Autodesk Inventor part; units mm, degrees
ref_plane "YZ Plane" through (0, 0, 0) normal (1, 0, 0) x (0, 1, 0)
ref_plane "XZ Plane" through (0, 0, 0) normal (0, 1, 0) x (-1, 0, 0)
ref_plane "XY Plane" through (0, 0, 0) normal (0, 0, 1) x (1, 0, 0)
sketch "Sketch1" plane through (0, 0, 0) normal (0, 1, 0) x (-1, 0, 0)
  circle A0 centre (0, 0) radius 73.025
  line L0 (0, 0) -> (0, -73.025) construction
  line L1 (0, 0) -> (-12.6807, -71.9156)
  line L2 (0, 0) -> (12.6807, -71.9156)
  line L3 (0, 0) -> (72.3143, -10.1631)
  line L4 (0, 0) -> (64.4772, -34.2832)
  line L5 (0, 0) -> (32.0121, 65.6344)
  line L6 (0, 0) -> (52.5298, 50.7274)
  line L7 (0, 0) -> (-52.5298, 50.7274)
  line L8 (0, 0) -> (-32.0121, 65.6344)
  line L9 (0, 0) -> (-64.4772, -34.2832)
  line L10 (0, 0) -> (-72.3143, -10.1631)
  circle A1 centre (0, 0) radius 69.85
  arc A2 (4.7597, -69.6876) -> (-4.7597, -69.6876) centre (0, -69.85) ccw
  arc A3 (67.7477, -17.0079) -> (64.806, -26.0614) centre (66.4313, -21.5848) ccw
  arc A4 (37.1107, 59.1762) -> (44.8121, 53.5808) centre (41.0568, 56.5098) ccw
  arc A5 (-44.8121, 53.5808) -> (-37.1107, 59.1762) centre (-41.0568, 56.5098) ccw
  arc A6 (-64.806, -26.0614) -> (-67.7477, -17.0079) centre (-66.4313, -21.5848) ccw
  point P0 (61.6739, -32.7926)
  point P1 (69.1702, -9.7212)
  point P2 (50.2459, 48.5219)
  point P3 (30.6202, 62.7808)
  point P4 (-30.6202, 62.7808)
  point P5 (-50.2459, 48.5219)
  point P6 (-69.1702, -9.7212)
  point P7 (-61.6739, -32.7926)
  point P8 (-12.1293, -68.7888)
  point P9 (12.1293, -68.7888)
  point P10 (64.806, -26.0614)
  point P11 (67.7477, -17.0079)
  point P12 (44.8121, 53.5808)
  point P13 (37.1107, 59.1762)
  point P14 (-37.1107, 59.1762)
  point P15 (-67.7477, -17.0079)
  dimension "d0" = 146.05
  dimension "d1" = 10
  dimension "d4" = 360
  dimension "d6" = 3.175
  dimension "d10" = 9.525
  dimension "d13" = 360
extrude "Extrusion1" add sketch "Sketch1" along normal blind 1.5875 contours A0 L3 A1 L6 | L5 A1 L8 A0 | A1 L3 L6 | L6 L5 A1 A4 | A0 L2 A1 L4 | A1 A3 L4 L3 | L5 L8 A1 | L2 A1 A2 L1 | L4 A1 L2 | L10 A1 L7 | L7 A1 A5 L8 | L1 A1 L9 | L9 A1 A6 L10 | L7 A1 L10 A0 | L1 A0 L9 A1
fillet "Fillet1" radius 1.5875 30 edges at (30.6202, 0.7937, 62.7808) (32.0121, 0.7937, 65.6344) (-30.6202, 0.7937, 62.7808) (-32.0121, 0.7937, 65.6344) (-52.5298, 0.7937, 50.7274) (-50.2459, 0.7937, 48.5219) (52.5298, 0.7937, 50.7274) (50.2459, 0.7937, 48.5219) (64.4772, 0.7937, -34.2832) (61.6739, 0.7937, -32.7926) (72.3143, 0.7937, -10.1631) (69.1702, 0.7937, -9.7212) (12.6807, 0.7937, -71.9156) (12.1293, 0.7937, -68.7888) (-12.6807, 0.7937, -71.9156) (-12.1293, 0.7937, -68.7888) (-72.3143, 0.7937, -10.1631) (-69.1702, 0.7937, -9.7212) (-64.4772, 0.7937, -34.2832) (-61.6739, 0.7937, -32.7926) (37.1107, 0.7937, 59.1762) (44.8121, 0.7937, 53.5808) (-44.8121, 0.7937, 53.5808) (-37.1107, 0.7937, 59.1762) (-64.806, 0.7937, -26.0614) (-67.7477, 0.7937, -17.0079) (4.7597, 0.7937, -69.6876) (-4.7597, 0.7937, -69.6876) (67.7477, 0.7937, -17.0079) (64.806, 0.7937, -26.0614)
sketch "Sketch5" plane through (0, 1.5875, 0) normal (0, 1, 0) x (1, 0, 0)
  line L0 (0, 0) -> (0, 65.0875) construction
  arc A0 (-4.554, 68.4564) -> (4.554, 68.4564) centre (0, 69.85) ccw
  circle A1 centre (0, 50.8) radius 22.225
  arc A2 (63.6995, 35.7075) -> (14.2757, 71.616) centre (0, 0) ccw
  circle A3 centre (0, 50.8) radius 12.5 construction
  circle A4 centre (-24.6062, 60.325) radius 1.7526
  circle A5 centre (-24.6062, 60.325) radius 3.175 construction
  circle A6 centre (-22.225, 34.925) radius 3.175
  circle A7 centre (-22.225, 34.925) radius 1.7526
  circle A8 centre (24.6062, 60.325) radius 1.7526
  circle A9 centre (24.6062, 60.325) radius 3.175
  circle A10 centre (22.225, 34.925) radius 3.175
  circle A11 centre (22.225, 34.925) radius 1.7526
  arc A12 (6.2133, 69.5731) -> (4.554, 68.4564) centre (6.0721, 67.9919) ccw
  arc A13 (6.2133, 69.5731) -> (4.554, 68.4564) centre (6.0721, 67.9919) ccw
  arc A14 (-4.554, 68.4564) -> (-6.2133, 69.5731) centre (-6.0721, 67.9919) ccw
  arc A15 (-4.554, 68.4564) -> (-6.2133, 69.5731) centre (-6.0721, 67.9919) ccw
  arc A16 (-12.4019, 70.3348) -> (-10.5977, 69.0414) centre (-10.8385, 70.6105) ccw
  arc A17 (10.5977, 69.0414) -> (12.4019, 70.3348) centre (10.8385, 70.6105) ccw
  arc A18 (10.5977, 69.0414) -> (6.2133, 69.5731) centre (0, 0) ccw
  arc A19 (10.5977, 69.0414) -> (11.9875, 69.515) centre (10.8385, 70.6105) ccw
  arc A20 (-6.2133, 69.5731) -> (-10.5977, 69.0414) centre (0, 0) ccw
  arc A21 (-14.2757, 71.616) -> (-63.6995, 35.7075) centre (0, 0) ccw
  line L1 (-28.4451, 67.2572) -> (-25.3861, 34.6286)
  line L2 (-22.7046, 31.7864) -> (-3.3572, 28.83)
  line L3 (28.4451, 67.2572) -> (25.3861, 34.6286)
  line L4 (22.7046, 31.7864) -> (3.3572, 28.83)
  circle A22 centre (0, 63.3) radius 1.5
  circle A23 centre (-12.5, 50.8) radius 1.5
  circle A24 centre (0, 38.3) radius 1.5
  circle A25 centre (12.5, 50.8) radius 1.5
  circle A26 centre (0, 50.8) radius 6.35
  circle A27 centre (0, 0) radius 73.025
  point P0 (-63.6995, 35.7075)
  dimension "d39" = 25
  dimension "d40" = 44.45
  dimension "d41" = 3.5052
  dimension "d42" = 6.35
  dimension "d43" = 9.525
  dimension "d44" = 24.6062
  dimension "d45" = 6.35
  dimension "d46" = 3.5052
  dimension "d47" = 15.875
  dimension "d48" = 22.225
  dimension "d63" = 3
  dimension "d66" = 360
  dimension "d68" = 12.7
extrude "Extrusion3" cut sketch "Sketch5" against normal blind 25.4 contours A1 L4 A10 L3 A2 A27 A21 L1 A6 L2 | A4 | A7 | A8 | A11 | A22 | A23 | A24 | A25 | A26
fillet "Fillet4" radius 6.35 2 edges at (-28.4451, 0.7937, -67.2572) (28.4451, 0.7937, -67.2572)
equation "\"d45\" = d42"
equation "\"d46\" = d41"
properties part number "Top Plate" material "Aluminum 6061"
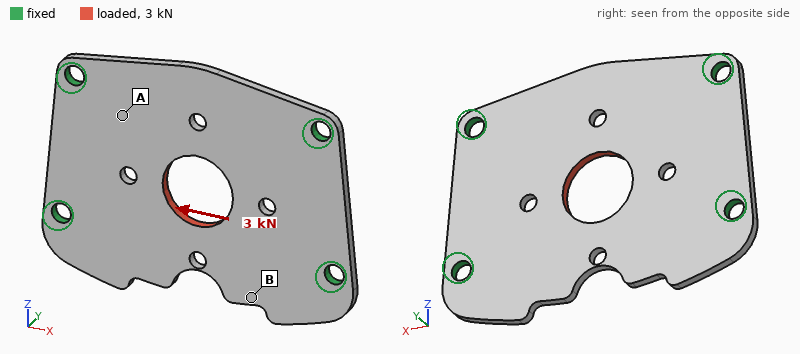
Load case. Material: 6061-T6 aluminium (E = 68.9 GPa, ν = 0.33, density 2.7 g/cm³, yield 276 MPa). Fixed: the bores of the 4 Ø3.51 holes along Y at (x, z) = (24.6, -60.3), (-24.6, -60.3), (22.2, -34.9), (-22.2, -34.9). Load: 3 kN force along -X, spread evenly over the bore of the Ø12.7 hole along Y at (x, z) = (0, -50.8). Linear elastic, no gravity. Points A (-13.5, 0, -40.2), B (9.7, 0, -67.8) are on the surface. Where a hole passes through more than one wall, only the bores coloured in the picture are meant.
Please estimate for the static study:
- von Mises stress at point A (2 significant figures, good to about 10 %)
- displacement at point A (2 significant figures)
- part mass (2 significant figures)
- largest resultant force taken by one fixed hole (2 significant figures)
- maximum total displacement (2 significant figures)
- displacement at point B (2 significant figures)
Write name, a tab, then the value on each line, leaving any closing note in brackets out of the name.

von Mises stress at point A	36 MPa
displacement at point A	6.4 µm
part mass	8.0 g
largest resultant force taken by one fixed hole	880 N
maximum total displacement	15 µm
displacement at point B	6.8 µm
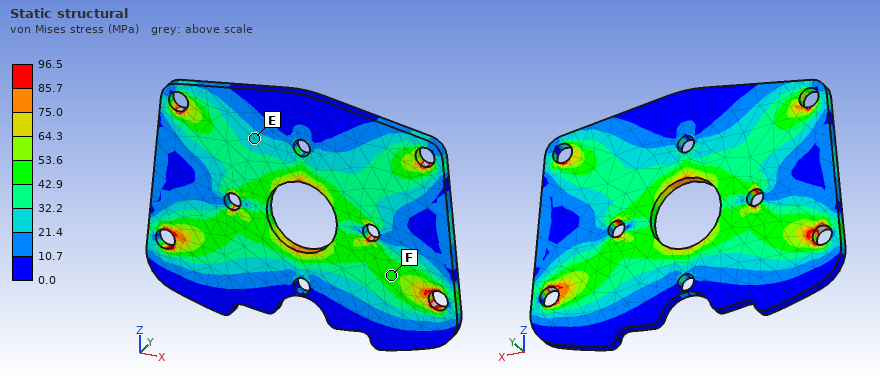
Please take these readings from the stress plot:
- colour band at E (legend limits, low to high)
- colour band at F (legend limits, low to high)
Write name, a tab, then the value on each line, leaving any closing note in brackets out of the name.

colour band at E	21.4 to 32.2 MPa
colour band at F	42.9 to 53.6 MPa
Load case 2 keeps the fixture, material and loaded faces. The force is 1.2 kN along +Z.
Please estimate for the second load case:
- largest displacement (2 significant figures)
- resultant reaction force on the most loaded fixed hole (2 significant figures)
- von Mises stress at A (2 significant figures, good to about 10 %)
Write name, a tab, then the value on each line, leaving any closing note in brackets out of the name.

largest displacement	16 µm
resultant reaction force on the most loaded fixed hole	420 N
von Mises stress at A	26 MPa
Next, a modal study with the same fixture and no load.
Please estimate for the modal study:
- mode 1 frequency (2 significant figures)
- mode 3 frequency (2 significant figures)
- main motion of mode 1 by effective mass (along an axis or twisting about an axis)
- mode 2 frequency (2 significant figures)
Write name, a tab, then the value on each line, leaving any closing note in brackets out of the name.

mode 1 frequency	3600 Hz
mode 3 frequency	7600 Hz
main motion of mode 1 by effective mass	along Y
mode 2 frequency	4800 Hz
